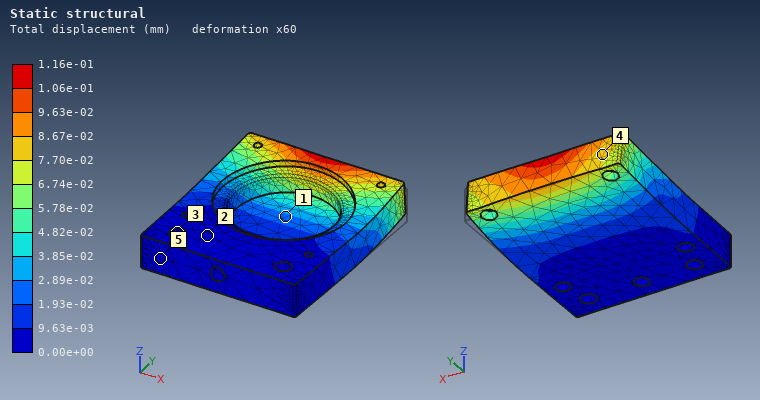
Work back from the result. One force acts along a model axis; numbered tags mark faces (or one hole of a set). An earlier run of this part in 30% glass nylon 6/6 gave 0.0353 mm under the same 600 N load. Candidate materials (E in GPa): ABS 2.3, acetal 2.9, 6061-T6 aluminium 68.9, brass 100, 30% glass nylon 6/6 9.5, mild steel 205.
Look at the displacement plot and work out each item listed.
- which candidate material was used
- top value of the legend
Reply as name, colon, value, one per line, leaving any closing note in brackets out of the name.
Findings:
which candidate material was used: acetal
top value of the legend: 1.16e-01 mm
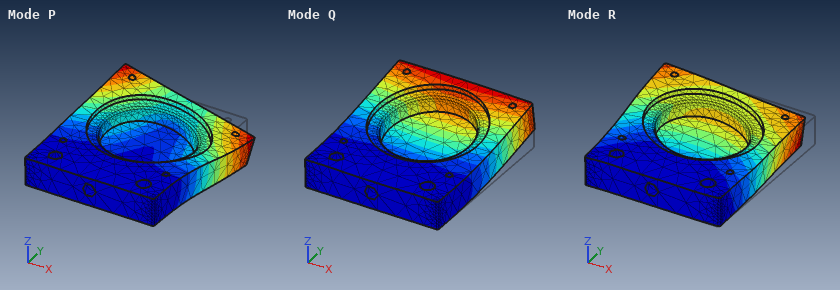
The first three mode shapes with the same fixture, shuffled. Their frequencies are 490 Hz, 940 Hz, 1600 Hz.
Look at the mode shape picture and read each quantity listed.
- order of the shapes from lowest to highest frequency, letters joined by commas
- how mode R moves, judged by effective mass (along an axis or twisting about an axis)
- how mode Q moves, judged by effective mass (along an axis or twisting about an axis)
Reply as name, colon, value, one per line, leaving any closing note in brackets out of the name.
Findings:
order of the shapes from lowest to highest frequency, letters joined by commas: Q, P, R
how mode R moves, judged by effective mass: along X
how mode Q moves, judged by effective mass: along Z
